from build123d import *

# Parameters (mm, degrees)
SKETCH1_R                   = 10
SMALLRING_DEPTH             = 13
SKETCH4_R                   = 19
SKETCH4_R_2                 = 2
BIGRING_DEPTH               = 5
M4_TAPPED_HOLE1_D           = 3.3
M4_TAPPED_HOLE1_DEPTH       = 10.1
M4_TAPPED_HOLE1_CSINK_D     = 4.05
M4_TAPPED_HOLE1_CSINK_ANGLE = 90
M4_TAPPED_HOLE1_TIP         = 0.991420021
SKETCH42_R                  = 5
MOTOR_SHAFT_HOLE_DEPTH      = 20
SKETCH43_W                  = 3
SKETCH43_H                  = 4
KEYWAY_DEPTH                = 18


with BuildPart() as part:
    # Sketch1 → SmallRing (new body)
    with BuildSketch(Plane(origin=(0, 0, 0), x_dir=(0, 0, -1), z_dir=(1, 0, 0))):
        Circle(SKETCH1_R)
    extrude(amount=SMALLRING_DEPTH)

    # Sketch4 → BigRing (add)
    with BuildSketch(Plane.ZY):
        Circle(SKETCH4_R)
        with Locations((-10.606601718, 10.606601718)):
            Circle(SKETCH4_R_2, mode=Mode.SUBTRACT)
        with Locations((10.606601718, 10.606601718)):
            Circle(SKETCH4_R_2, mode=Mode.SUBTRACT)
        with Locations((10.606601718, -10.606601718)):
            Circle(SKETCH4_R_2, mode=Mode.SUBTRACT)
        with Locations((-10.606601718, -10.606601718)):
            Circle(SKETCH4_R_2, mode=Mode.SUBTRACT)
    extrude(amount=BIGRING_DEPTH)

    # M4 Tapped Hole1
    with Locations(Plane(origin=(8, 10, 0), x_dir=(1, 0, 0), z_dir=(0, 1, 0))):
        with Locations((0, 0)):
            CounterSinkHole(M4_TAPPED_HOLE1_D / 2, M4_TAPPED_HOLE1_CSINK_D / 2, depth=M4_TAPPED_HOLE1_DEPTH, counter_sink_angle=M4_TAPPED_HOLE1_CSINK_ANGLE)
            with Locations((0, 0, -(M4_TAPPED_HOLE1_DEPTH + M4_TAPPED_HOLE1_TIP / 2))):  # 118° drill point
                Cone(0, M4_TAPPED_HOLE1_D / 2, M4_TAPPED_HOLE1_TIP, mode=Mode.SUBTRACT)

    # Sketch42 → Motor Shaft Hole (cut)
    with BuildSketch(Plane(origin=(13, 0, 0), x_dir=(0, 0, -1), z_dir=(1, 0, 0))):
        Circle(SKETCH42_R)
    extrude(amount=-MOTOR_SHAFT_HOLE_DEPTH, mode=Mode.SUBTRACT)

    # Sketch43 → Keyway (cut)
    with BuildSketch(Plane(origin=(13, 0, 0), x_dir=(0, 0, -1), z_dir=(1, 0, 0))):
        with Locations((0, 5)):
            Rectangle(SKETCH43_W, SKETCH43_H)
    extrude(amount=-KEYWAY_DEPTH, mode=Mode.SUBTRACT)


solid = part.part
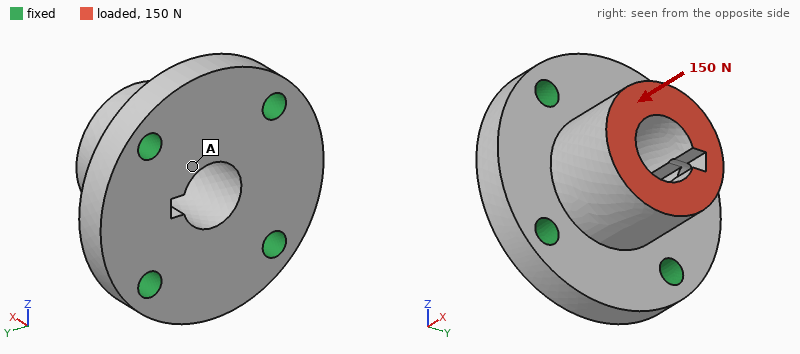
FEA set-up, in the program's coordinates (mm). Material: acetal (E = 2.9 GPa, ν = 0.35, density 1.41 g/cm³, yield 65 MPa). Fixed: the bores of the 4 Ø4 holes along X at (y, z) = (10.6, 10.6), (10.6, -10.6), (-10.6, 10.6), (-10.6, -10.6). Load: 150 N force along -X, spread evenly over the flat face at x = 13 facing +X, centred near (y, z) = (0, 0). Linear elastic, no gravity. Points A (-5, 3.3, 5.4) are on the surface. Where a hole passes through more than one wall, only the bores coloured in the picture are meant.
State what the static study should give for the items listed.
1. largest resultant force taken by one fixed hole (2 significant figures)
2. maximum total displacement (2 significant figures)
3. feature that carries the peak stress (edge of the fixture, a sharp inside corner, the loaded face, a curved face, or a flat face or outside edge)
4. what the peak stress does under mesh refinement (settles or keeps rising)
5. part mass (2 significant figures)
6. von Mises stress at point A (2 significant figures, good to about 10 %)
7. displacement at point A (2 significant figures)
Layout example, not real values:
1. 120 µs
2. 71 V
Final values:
1. 40 N
2. 10 µm
3. edge of the fixture
4. keeps rising
5. 11 g
6. 0.63 MPa
7. 7.1 µm
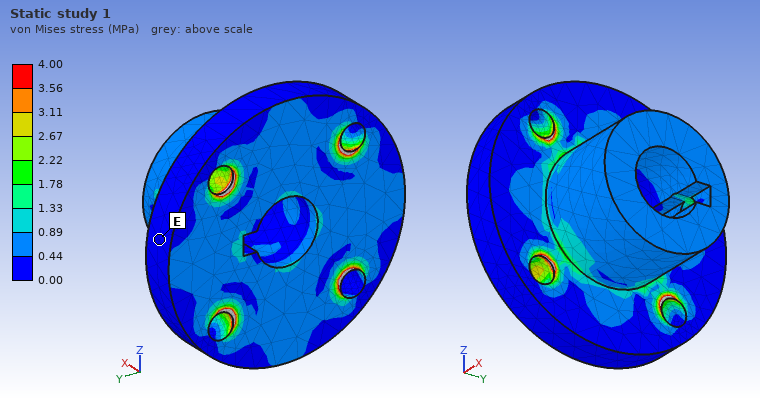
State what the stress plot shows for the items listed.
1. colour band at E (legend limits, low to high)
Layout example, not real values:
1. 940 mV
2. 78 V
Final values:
1. 0.00 to 0.44 MPa
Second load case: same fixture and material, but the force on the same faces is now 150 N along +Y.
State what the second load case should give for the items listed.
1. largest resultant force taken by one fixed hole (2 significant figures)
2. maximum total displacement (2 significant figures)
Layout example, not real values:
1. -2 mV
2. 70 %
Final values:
1. 72 N
2. 45 µm
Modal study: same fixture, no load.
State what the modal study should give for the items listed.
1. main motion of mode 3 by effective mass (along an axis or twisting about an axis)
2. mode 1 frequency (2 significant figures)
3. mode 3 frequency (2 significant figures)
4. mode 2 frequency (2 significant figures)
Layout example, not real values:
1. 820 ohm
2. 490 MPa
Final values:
1. along X
2. 7100 Hz
3. 9000 Hz
4. 7200 Hz
